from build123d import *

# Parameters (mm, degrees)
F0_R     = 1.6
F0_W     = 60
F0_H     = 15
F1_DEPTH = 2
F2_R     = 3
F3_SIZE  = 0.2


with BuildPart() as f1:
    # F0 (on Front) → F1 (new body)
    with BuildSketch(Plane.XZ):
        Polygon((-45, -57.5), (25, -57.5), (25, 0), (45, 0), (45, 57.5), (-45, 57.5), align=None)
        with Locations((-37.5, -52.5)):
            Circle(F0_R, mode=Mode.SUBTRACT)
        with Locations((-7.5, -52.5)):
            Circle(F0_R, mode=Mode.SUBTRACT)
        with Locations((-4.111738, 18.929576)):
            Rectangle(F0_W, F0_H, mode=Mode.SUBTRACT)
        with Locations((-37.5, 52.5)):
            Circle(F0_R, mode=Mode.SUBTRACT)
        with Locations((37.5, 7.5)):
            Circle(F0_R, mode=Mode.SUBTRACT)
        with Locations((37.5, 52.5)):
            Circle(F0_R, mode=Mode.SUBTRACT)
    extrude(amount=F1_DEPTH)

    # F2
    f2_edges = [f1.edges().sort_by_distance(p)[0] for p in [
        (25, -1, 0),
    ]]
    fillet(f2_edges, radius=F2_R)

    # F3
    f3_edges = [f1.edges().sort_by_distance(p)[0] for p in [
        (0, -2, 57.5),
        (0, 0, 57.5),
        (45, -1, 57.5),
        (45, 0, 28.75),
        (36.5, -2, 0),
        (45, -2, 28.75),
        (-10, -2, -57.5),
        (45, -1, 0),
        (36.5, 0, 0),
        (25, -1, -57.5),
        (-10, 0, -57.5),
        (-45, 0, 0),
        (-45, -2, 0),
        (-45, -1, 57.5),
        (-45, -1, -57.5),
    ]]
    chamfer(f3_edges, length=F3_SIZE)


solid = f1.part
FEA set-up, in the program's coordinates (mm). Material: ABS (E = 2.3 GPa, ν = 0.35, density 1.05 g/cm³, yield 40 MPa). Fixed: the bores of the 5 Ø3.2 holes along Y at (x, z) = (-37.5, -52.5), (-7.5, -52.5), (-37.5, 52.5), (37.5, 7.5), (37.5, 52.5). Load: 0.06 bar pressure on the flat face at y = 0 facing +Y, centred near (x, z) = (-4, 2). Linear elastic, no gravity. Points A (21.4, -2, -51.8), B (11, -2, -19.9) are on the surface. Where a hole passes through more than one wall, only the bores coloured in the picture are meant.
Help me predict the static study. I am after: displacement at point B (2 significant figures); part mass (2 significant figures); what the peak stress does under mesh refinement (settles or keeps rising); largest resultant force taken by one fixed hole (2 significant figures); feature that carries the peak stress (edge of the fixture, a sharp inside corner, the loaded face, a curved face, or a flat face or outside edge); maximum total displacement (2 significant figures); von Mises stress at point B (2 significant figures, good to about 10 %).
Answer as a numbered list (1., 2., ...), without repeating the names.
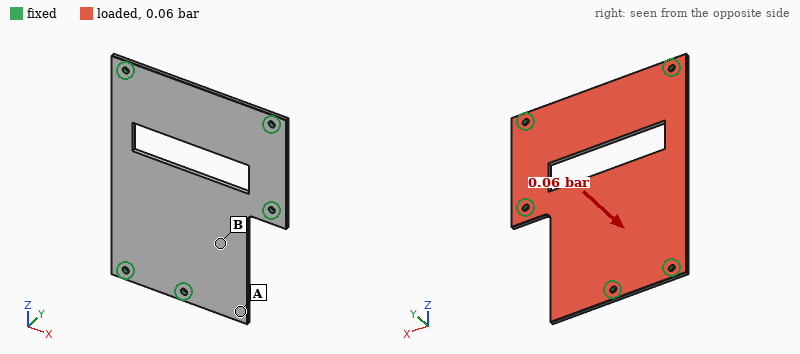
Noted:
1. 0.61 mm
2. 17 g
3. keeps rising
4. 12 N
5. edge of the fixture
6. 1.4 mm
7. 3.0 MPa
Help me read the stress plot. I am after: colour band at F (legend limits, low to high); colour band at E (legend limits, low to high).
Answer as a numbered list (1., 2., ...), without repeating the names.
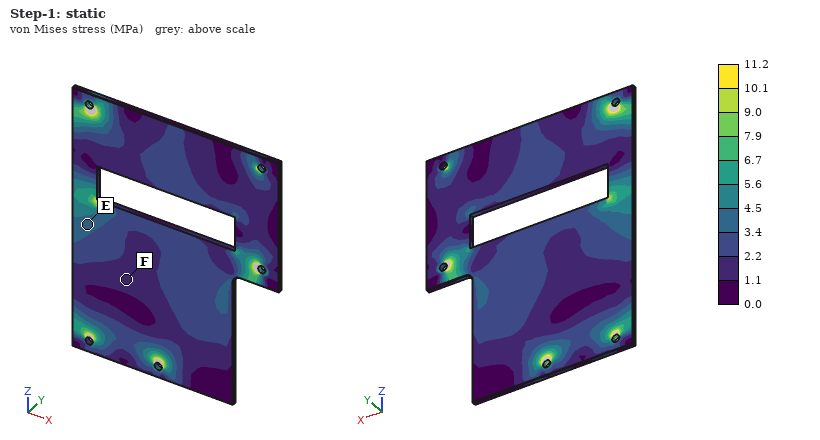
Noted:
1. 1.1 to 2.2 MPa
2. 3.4 to 4.5 MPa
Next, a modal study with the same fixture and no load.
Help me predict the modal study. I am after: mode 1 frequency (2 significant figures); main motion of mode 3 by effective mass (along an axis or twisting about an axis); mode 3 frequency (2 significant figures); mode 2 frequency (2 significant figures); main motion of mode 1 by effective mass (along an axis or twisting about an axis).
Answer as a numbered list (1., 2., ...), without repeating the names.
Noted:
1. 270 Hz
2. along Y
3. 470 Hz
4. 440 Hz
5. along Y
